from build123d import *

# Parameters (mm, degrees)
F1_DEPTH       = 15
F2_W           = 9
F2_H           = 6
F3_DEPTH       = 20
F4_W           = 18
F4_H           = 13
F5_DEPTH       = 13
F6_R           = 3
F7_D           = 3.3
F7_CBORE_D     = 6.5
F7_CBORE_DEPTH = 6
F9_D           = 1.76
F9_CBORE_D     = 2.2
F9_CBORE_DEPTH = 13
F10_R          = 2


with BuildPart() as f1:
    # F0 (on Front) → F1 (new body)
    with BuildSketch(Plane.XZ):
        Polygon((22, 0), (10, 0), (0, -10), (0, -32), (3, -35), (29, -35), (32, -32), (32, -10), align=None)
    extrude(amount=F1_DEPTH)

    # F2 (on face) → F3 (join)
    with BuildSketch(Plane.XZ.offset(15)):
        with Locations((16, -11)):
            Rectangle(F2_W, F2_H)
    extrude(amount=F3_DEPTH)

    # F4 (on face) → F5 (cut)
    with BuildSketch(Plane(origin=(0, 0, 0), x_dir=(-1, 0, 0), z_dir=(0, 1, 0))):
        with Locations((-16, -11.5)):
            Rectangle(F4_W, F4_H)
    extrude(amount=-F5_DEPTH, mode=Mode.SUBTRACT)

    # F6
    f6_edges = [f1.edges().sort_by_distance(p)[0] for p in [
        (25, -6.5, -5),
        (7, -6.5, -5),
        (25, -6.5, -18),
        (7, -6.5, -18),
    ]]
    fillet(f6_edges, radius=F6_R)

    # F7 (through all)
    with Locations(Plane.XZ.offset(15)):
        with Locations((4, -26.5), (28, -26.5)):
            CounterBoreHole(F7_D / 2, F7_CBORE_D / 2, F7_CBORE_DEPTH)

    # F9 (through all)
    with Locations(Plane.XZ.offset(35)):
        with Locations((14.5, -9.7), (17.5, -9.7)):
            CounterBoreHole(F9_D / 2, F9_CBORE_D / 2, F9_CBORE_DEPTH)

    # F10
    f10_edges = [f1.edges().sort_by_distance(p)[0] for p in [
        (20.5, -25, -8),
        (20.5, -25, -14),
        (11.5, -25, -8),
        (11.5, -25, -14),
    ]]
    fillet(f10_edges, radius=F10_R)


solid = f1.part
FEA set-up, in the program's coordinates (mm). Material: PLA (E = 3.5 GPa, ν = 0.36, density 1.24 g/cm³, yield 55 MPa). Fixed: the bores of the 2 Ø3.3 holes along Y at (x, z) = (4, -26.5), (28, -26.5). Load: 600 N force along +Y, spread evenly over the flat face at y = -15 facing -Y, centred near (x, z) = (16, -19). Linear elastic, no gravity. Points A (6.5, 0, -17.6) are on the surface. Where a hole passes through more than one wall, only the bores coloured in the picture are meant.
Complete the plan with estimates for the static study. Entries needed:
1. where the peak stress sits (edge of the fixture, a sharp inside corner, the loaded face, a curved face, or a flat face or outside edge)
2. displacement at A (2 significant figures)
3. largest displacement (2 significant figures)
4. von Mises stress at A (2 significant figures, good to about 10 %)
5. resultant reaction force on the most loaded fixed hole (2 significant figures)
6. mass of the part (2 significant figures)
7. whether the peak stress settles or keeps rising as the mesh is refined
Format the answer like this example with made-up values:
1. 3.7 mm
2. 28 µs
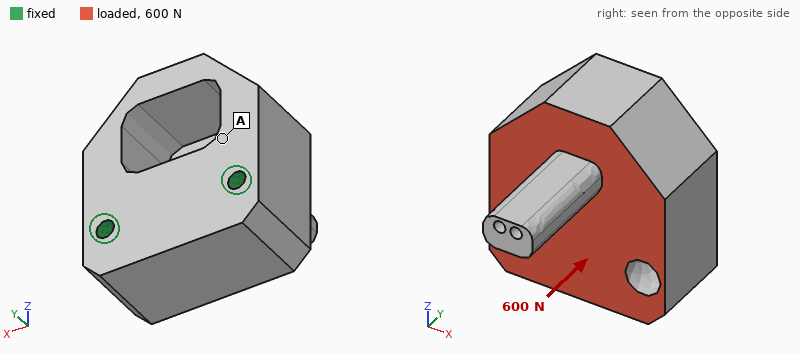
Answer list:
1. edge of the fixture
2. 0.044 mm
3. 0.20 mm
4. 5.0 MPa
5. 310 N
6. 16 g
7. keeps rising
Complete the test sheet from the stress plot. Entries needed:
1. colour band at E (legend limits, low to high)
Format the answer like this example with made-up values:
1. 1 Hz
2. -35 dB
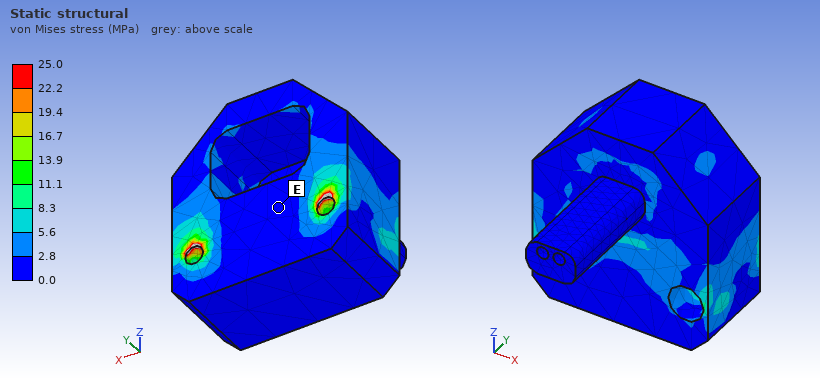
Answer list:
1. 0.0 to 2.8 MPa
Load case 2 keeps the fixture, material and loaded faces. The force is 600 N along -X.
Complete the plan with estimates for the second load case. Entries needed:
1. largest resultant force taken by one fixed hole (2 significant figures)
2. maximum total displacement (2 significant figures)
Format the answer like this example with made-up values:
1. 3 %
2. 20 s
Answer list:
1. 420 N
2. 51 µm
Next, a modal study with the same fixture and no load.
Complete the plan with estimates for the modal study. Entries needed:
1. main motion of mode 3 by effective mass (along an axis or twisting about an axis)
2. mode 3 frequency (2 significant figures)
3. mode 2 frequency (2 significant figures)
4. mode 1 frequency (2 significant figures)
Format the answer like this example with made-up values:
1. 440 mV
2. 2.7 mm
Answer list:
1. along Y
2. 3600 Hz
3. 3000 Hz
4. 2300 Hz
